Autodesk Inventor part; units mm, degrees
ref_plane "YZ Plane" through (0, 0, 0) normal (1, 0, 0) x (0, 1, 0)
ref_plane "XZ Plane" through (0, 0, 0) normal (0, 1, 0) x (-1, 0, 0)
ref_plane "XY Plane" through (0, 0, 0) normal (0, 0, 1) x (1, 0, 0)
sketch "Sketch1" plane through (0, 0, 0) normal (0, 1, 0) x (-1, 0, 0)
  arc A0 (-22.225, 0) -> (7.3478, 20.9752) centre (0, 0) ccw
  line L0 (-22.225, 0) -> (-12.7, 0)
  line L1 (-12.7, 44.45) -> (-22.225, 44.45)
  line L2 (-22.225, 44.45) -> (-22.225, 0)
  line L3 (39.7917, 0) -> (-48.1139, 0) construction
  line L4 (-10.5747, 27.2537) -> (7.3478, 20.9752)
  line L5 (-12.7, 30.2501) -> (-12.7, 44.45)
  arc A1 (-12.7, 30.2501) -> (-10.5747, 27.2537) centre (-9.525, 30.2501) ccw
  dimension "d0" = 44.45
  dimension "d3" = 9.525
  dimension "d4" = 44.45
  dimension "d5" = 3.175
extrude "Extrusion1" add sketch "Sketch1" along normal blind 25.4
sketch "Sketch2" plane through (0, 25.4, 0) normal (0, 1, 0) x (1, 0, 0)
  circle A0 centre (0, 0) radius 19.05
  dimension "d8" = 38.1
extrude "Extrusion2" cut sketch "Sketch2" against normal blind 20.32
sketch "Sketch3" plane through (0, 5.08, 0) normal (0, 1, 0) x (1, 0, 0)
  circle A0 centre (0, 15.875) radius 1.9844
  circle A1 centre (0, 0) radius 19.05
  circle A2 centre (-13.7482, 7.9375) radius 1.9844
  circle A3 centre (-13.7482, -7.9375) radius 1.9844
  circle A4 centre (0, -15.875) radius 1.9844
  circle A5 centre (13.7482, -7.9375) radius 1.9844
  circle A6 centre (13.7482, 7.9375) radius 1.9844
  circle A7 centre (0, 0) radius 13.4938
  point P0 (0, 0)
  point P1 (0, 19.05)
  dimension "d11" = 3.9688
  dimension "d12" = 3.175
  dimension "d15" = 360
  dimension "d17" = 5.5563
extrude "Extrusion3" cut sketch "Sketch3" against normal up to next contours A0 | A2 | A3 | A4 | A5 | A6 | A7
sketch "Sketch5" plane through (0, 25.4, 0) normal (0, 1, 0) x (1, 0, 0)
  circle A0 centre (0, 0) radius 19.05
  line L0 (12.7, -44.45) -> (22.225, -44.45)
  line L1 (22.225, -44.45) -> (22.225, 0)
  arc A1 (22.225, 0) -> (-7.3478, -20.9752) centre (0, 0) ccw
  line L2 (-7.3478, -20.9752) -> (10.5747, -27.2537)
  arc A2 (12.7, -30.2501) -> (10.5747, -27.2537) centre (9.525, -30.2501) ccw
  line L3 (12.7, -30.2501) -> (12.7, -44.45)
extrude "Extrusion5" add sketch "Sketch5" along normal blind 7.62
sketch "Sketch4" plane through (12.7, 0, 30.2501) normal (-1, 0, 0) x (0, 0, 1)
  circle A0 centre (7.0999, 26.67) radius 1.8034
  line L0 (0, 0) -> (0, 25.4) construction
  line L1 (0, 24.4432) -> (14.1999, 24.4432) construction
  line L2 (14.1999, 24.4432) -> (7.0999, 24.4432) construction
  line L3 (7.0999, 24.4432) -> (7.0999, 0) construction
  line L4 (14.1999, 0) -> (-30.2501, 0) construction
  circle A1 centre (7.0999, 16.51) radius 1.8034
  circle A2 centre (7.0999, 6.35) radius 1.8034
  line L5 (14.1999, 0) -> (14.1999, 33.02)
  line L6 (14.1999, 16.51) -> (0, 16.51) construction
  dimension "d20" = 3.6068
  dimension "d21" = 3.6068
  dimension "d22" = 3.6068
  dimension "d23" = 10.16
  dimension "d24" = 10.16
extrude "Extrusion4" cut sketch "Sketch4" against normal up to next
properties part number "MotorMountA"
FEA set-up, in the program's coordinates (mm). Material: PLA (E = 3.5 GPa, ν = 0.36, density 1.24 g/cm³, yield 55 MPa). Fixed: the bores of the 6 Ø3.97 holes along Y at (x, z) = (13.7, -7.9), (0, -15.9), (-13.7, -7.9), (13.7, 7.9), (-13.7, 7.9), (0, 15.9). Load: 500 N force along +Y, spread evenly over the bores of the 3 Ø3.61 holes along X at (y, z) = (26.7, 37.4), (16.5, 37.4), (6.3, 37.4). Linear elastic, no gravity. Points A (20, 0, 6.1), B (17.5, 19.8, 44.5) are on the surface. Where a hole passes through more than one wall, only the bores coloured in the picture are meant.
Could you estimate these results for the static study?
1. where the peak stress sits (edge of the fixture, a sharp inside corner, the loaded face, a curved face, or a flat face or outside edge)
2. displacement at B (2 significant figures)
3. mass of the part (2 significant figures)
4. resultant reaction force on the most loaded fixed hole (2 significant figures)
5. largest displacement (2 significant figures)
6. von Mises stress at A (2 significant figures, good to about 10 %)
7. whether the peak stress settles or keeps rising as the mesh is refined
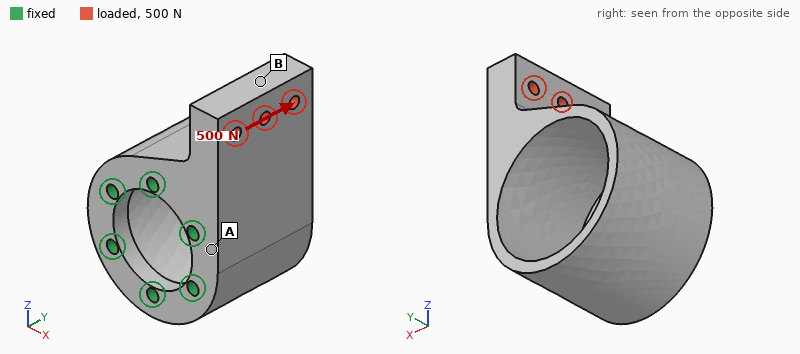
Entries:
edge of the fixture
0.41 mm
35 g
520 N
0.49 mm
8.1 MPa
keeps rising
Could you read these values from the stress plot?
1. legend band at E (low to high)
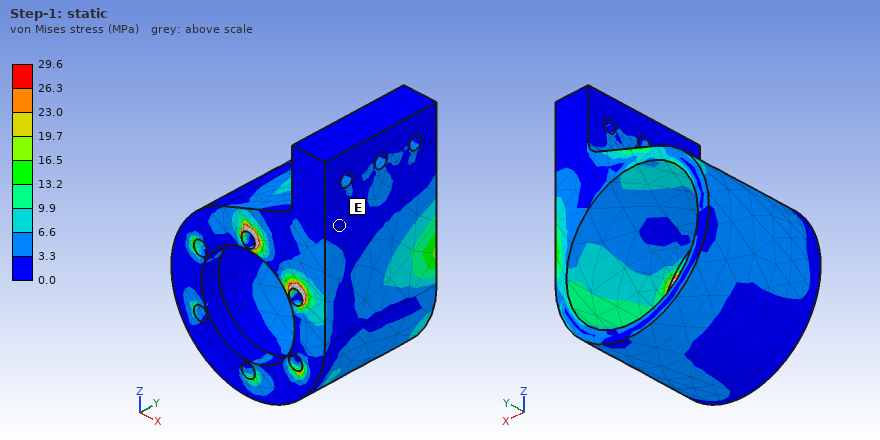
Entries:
0.0 to 3.3 MPa
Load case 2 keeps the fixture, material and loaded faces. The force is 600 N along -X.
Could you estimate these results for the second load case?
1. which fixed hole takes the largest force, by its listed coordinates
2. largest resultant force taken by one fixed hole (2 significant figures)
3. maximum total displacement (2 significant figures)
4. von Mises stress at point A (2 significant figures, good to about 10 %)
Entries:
(0, 15.9)
650 N
0.37 mm
6.5 MPa
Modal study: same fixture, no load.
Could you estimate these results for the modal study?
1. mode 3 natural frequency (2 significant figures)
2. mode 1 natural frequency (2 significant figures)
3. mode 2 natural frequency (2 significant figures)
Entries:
3000 Hz
1700 Hz
2900 Hz
